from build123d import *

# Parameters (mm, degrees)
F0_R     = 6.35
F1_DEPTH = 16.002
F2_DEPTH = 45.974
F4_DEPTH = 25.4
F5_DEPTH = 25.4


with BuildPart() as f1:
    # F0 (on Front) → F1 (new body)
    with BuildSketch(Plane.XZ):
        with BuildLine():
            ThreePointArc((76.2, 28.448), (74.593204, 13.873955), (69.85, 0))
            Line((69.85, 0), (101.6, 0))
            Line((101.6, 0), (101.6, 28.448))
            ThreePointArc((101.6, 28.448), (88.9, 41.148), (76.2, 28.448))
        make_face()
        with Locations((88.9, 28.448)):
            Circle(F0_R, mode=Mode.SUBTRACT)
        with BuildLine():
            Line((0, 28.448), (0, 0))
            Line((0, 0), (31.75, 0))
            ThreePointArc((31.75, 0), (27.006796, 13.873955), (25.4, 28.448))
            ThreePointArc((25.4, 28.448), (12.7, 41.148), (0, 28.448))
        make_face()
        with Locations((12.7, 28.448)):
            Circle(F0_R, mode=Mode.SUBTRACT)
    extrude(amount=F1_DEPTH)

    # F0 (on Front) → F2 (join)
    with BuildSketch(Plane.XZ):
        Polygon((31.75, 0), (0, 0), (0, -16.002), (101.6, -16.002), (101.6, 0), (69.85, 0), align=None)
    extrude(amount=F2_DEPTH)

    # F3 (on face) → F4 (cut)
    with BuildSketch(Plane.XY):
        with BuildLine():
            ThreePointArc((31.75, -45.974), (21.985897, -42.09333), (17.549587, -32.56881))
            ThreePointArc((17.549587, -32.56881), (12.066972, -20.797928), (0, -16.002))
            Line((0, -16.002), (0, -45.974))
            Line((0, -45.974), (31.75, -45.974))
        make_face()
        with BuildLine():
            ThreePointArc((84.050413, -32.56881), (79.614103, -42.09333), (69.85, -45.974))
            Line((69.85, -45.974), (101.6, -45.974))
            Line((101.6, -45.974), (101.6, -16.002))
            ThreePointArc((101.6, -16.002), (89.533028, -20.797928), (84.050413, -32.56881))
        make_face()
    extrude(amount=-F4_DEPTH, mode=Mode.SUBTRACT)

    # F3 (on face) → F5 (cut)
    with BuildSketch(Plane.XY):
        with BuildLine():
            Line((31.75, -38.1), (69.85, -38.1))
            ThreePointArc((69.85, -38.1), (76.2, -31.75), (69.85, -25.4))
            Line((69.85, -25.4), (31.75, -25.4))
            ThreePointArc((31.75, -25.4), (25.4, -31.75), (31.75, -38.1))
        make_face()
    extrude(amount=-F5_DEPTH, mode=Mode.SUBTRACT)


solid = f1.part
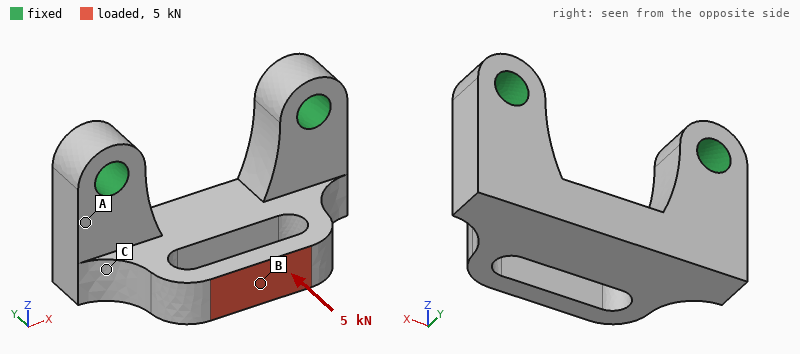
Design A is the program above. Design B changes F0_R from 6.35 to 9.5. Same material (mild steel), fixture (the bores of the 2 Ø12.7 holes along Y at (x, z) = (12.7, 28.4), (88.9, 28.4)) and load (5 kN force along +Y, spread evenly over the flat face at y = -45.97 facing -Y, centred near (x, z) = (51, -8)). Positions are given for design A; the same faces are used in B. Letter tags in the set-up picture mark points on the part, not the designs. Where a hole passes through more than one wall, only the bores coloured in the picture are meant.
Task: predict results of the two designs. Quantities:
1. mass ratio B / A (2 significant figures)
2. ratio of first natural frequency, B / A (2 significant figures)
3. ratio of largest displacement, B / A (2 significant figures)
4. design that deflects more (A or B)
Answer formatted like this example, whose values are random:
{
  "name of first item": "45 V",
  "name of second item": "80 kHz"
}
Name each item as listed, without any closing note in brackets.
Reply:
{
  "mass ratio B / A": "0.94",
  "ratio of first natural frequency, B / A": "1.1",
  "ratio of largest displacement, B / A": "0.87",
  "design that deflects more": "A"
}
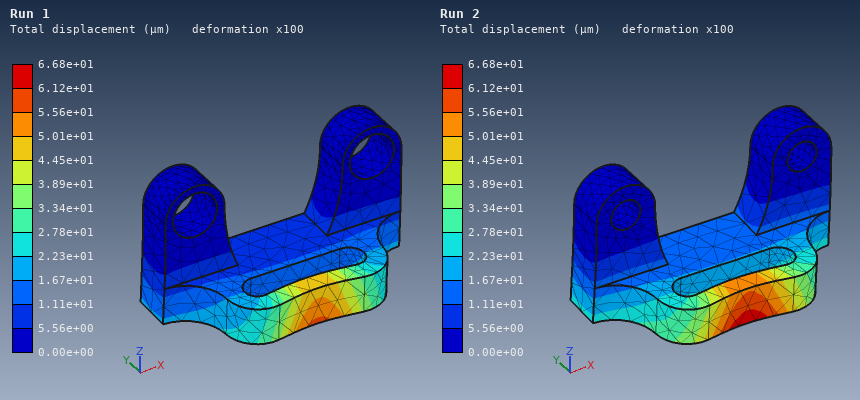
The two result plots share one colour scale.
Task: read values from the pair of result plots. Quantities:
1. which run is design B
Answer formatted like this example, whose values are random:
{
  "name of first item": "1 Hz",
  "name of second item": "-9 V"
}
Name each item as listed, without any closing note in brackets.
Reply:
{
  "which run is design B": "Run 1"
}
